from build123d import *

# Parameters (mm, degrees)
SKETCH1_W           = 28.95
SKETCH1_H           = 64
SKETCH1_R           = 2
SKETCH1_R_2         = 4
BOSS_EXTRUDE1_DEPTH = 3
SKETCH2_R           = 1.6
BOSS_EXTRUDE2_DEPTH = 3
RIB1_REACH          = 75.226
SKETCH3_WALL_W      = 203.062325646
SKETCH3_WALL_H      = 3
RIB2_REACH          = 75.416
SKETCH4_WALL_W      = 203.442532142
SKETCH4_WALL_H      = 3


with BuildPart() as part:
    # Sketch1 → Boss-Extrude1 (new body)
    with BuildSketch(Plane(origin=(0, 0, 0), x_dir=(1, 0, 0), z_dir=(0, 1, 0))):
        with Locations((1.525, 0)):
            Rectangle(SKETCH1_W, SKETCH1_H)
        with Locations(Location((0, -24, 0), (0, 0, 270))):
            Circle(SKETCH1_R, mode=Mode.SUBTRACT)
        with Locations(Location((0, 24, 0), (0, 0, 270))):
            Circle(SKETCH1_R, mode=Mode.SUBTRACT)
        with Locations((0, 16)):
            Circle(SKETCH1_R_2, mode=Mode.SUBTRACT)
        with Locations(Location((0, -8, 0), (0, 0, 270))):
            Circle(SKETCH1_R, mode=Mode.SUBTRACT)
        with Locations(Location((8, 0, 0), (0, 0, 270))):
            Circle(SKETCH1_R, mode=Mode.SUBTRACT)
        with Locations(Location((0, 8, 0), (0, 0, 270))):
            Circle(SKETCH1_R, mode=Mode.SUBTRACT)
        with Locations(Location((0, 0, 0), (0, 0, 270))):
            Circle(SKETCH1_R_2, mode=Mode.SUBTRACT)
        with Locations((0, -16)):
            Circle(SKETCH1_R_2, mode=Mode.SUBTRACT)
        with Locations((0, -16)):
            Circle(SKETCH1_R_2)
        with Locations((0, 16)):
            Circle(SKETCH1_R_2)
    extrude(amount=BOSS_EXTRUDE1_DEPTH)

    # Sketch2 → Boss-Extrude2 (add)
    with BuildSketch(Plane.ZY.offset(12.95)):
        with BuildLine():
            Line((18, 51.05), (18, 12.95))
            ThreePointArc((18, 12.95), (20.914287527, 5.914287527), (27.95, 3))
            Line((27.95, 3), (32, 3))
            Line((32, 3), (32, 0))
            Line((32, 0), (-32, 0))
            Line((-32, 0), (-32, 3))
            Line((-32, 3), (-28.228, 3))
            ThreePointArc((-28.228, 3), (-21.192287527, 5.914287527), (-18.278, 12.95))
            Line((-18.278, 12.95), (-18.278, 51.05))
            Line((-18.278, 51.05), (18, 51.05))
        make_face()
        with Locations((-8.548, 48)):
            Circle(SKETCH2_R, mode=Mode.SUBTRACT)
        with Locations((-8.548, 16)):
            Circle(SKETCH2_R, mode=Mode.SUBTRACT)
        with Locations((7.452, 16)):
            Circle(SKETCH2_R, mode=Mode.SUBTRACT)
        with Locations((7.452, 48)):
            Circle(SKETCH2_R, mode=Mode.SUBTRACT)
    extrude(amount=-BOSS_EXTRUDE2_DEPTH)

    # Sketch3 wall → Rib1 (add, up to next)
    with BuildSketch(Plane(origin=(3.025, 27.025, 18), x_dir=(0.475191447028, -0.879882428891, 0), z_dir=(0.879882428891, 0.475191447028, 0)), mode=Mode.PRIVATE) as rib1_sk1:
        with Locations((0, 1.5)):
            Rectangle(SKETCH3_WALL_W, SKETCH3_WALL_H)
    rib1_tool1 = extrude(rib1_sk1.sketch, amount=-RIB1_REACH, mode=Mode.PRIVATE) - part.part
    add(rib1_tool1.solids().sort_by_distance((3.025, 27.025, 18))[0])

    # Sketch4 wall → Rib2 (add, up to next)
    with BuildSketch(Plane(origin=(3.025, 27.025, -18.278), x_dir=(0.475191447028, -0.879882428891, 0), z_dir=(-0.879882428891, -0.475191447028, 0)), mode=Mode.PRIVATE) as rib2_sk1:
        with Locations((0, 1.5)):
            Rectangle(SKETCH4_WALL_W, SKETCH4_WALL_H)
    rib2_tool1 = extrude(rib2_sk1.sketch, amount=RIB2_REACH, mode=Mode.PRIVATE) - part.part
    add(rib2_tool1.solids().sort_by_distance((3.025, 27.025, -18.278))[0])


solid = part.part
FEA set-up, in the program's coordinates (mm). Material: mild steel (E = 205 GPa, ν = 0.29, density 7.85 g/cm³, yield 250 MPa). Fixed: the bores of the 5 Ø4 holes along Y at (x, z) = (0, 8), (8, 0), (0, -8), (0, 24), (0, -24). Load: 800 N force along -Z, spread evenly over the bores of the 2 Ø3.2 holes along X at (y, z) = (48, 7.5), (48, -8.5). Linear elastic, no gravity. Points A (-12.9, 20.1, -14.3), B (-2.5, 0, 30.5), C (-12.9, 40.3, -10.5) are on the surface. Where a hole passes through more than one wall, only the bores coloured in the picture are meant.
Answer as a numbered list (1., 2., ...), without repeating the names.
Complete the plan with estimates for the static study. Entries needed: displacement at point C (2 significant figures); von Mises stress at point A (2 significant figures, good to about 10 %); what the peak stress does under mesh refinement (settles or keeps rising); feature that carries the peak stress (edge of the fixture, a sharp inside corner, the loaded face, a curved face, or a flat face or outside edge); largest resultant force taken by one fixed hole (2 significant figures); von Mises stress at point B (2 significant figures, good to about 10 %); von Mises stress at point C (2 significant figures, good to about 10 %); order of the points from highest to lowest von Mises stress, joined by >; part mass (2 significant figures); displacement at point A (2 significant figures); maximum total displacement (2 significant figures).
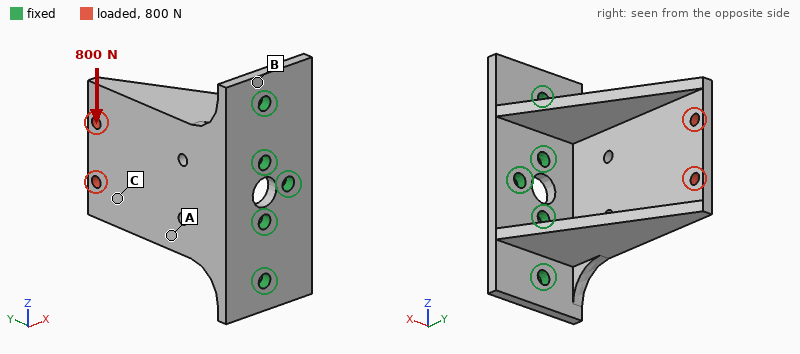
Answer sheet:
1. 37 µm
2. 25 MPa
3. keeps rising
4. edge of the fixture
5. 830 N
6. 49 MPa
7. 14 MPa
8. B > A > C
9. 110 g
10. 22 µm
11. 64 µm
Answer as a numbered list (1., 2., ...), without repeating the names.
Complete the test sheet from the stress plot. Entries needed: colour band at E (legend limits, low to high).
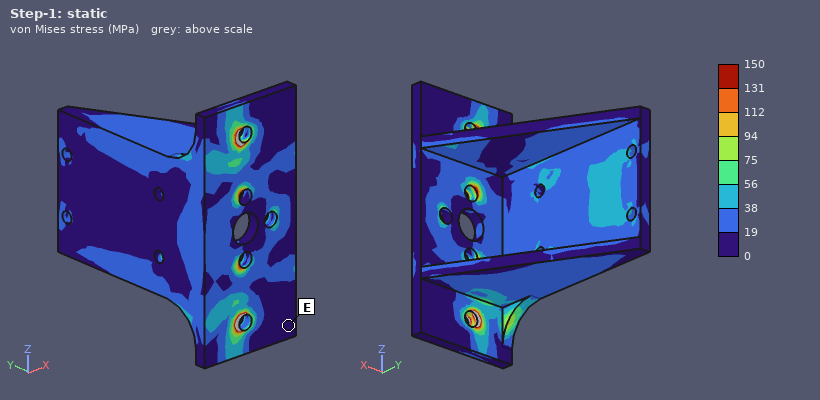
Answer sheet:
1. 0 to 19 MPa
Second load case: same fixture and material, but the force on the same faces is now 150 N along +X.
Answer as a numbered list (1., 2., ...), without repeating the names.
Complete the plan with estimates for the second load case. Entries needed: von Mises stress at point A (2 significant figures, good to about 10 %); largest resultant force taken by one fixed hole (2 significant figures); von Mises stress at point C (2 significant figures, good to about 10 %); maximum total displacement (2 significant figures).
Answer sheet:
1. 6.8 MPa
2. 100 N
3. 15 MPa
4. 34 µm
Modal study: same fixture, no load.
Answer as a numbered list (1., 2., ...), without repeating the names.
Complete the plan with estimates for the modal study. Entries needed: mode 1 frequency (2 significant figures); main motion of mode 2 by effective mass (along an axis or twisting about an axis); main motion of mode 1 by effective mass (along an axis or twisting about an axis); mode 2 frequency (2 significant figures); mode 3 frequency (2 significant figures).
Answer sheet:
1. 2600 Hz
2. along Z
3. along X
4. 3500 Hz
5. 8700 Hz
